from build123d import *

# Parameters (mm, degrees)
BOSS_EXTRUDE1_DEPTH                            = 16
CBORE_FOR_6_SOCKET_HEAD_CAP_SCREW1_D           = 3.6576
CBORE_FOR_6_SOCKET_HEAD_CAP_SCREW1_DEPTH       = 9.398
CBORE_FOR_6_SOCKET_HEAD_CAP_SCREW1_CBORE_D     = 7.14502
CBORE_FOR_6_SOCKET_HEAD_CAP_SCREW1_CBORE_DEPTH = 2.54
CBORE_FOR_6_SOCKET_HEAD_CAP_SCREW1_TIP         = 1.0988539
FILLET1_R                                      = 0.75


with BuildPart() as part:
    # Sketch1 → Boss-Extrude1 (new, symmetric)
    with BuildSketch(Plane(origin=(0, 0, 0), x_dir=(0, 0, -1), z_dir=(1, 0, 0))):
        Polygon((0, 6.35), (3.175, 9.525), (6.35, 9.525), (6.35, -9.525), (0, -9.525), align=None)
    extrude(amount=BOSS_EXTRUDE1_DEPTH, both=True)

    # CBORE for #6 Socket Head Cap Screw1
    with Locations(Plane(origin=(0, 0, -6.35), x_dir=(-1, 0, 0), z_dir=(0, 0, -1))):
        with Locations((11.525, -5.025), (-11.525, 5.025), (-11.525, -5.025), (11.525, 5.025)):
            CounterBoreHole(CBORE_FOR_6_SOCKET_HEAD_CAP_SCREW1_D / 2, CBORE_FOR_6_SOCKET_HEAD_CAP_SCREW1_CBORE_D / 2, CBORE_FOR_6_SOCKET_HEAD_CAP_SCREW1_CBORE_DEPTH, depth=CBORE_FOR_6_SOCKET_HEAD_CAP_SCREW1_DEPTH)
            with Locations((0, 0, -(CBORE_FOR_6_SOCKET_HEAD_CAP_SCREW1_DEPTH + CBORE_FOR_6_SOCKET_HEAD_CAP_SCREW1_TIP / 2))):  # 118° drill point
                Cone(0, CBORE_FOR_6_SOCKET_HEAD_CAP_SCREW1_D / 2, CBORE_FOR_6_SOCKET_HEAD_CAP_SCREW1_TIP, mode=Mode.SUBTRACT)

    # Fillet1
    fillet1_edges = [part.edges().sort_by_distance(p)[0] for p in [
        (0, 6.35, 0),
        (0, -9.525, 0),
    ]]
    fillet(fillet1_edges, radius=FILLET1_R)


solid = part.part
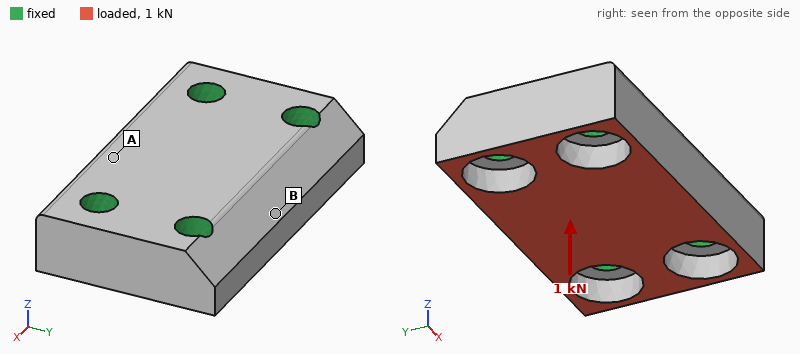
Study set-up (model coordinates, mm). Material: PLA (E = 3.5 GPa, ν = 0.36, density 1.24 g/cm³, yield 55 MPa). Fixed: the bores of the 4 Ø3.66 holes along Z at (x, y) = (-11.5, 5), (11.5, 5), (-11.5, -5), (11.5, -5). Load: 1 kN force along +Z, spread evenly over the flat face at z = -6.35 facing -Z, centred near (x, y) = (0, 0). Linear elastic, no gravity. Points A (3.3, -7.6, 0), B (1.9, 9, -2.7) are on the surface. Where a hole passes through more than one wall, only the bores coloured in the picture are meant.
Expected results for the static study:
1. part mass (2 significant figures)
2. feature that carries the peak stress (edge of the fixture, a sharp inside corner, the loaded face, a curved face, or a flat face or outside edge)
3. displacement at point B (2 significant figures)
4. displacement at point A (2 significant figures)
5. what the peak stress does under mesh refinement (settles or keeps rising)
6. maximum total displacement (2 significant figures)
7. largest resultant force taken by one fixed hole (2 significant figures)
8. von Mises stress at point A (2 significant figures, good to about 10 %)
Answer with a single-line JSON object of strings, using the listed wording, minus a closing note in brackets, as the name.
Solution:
{"part mass": "3.9 g", "feature that carries the peak stress": "edge of the fixture", "displacement at point B": "60 µm", "displacement at point A": "44 µm", "what the peak stress does under mesh refinement": "keeps rising", "maximum total displacement": "66 µm", "largest resultant force taken by one fixed hole": "270 N", "von Mises stress at point A": "6.2 MPa"}
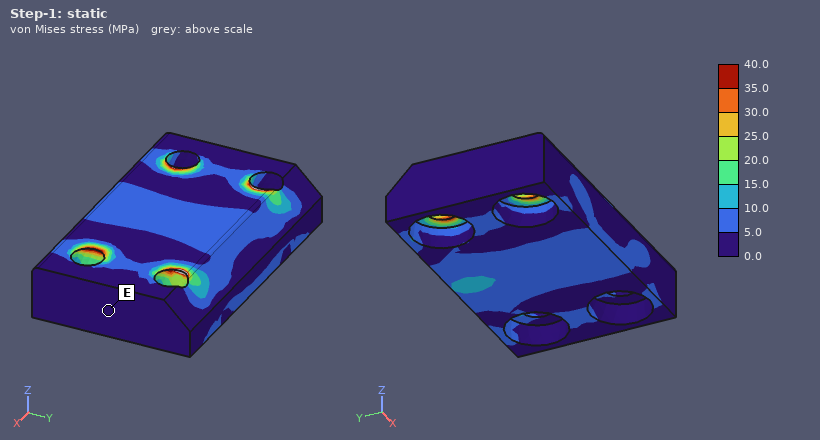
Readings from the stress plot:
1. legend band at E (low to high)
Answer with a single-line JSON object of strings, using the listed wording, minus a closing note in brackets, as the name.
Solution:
{"legend band at E": "0.0 to 5.0 MPa"}
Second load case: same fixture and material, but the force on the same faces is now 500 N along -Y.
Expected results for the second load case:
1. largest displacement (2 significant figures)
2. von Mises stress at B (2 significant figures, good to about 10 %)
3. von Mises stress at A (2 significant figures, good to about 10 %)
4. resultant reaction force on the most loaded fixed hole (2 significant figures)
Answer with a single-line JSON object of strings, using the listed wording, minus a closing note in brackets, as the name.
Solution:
{"largest displacement": "41 µm", "von Mises stress at B": "2.9 MPa", "von Mises stress at A": "2.9 MPa", "resultant reaction force on the most loaded fixed hole": "170 N"}
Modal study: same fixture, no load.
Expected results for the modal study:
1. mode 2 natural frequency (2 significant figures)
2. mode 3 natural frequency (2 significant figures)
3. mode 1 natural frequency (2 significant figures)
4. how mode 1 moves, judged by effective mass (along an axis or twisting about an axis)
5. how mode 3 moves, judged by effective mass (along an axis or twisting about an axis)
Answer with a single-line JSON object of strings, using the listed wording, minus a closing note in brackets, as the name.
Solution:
{"mode 2 natural frequency": "15 kHz", "mode 3 natural frequency": "19 kHz", "mode 1 natural frequency": "13 kHz", "how mode 1 moves, judged by effective mass": "along Z", "how mode 3 moves, judged by effective mass": "along Y"}
